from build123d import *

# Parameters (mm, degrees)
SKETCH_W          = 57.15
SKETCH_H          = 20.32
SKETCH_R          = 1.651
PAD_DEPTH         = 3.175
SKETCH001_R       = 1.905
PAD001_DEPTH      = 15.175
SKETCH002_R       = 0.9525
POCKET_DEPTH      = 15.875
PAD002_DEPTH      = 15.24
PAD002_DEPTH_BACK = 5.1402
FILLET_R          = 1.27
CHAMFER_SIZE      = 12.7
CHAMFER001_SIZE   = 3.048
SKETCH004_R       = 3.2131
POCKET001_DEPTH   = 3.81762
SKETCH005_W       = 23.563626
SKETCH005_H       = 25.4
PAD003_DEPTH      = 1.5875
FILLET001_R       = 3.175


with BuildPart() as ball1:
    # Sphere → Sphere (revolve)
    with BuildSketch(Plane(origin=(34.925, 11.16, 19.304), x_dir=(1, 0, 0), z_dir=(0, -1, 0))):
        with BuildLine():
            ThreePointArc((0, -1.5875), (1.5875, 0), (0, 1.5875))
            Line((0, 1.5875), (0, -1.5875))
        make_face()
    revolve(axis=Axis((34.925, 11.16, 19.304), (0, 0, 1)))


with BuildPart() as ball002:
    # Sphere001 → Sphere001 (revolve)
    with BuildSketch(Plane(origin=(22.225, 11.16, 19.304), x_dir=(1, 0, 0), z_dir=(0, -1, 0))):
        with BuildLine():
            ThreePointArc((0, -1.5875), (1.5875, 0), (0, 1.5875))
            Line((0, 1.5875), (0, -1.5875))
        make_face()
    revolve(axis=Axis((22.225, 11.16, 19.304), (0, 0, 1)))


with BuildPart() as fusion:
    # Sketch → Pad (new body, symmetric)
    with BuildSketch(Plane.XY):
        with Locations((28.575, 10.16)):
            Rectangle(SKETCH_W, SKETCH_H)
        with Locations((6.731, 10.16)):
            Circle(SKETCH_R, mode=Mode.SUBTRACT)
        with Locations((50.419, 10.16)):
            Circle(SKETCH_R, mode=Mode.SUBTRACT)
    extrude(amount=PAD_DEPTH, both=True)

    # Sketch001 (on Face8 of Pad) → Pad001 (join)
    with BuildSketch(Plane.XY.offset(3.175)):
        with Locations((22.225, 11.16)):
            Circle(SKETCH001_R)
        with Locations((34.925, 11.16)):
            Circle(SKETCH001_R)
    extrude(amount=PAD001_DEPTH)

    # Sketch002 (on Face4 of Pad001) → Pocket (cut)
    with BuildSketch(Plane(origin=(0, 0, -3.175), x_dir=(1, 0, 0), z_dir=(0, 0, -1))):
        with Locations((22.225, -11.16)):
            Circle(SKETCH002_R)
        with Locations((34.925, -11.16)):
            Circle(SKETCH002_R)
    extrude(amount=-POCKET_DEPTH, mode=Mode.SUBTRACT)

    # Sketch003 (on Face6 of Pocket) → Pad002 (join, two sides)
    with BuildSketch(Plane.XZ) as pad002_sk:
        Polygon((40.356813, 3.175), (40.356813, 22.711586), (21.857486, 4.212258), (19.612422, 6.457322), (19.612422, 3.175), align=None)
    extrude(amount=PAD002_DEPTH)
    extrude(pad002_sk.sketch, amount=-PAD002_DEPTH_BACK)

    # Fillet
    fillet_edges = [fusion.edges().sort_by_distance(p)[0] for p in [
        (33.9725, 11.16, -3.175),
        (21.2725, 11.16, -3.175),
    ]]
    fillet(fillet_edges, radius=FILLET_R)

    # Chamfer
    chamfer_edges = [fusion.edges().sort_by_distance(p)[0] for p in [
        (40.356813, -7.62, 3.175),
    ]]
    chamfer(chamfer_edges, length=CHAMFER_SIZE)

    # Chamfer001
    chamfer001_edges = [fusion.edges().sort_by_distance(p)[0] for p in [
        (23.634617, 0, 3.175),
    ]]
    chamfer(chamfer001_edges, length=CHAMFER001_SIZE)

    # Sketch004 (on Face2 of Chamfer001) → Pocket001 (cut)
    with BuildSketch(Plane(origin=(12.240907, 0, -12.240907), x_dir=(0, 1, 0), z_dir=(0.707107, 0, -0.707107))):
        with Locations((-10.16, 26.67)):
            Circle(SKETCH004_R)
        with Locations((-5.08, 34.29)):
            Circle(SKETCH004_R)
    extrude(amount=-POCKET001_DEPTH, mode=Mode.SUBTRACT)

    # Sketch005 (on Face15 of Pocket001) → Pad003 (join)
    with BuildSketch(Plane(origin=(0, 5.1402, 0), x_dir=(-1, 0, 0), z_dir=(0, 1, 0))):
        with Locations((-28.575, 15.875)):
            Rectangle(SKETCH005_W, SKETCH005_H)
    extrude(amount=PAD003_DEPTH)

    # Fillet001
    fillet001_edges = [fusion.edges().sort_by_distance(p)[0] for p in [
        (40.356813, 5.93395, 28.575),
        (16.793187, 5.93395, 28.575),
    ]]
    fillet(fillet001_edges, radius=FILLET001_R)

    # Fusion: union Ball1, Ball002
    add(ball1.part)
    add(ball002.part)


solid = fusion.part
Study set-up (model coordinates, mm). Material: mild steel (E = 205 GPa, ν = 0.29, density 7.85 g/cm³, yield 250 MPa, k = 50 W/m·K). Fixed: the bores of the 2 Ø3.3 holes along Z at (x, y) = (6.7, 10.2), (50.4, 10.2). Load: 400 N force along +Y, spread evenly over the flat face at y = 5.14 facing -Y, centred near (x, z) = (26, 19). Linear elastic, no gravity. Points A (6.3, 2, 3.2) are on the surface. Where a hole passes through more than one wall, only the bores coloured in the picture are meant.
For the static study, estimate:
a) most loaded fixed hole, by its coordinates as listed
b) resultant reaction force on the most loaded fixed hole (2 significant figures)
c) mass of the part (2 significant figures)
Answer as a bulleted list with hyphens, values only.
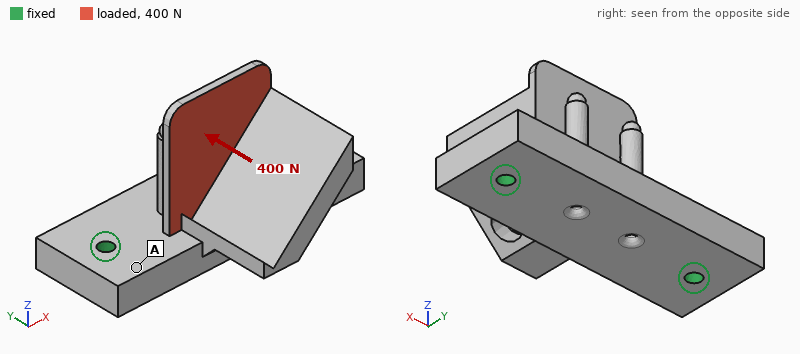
- (6.7, 10.2)
- 220 N
- 87 g
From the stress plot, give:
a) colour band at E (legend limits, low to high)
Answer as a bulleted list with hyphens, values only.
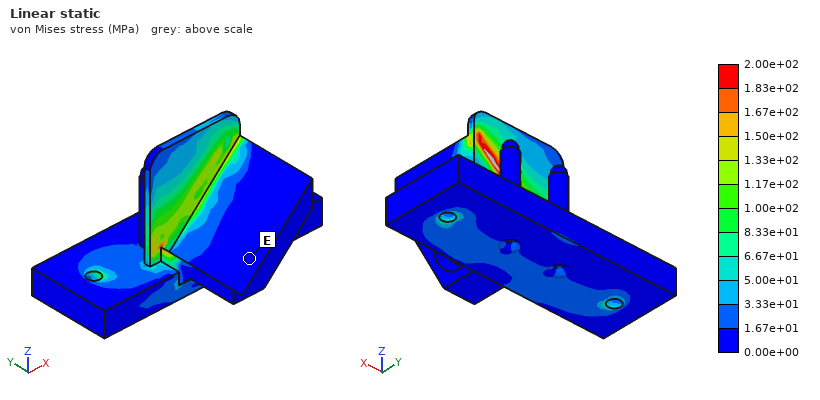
- 0.00e+00 to 1.67e+01 MPa
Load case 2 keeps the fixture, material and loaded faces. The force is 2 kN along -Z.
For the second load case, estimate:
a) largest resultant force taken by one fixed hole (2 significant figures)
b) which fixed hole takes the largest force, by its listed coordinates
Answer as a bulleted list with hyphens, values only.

- 1.2 kN
- (6.7, 10.2)
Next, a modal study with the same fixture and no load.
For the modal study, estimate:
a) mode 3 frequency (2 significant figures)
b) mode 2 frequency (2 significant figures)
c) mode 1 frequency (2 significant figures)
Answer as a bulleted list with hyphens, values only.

- 8300 Hz
- 6100 Hz
- 4100 Hz
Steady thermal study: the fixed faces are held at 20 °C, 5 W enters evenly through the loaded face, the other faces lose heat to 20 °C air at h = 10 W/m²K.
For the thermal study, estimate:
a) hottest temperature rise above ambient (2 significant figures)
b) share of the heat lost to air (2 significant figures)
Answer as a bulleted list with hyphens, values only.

- 35 K
- 9.2 %
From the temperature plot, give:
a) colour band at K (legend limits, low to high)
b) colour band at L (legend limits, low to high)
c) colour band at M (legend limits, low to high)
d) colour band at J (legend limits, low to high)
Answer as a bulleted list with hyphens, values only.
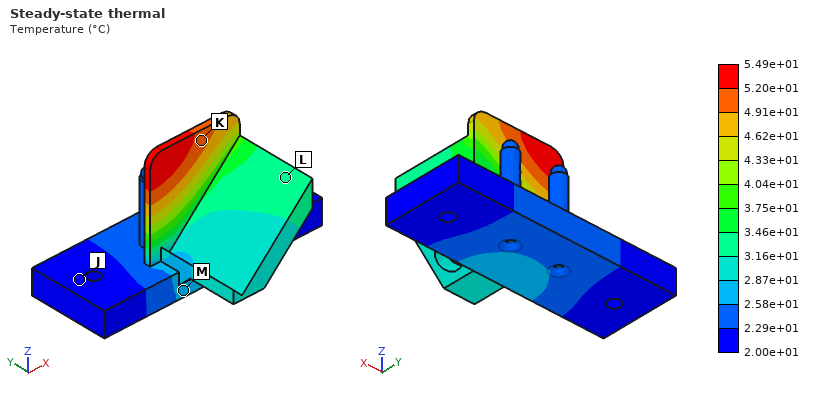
- 4.91e+01 to 5.20e+01 °C
- 3.16e+01 to 3.46e+01 °C
- 2.58e+01 to 2.87e+01 °C
- 2.00e+01 to 2.29e+01 °C
